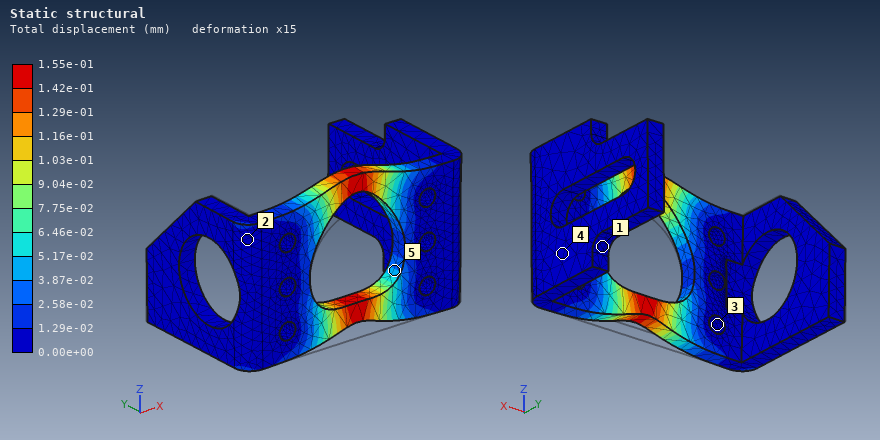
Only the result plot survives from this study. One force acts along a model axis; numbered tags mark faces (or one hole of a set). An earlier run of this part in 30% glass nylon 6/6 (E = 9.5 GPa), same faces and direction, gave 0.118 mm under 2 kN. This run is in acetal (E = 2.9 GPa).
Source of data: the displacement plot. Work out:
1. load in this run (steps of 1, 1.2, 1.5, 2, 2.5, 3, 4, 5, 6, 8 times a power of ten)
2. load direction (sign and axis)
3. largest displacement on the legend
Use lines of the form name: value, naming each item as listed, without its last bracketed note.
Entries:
load in this run: 800 N
load direction: +Z
largest displacement on the legend: 1.55e-01 mm
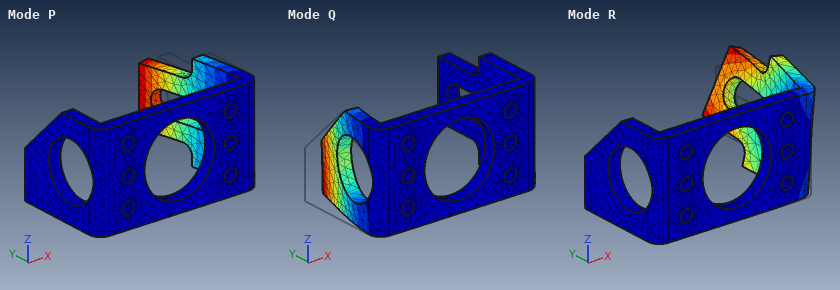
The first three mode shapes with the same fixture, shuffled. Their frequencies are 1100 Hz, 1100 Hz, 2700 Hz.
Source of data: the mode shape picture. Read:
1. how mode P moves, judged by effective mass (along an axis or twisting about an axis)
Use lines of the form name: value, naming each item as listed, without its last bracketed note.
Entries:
how mode P moves, judged by effective mass: along X
